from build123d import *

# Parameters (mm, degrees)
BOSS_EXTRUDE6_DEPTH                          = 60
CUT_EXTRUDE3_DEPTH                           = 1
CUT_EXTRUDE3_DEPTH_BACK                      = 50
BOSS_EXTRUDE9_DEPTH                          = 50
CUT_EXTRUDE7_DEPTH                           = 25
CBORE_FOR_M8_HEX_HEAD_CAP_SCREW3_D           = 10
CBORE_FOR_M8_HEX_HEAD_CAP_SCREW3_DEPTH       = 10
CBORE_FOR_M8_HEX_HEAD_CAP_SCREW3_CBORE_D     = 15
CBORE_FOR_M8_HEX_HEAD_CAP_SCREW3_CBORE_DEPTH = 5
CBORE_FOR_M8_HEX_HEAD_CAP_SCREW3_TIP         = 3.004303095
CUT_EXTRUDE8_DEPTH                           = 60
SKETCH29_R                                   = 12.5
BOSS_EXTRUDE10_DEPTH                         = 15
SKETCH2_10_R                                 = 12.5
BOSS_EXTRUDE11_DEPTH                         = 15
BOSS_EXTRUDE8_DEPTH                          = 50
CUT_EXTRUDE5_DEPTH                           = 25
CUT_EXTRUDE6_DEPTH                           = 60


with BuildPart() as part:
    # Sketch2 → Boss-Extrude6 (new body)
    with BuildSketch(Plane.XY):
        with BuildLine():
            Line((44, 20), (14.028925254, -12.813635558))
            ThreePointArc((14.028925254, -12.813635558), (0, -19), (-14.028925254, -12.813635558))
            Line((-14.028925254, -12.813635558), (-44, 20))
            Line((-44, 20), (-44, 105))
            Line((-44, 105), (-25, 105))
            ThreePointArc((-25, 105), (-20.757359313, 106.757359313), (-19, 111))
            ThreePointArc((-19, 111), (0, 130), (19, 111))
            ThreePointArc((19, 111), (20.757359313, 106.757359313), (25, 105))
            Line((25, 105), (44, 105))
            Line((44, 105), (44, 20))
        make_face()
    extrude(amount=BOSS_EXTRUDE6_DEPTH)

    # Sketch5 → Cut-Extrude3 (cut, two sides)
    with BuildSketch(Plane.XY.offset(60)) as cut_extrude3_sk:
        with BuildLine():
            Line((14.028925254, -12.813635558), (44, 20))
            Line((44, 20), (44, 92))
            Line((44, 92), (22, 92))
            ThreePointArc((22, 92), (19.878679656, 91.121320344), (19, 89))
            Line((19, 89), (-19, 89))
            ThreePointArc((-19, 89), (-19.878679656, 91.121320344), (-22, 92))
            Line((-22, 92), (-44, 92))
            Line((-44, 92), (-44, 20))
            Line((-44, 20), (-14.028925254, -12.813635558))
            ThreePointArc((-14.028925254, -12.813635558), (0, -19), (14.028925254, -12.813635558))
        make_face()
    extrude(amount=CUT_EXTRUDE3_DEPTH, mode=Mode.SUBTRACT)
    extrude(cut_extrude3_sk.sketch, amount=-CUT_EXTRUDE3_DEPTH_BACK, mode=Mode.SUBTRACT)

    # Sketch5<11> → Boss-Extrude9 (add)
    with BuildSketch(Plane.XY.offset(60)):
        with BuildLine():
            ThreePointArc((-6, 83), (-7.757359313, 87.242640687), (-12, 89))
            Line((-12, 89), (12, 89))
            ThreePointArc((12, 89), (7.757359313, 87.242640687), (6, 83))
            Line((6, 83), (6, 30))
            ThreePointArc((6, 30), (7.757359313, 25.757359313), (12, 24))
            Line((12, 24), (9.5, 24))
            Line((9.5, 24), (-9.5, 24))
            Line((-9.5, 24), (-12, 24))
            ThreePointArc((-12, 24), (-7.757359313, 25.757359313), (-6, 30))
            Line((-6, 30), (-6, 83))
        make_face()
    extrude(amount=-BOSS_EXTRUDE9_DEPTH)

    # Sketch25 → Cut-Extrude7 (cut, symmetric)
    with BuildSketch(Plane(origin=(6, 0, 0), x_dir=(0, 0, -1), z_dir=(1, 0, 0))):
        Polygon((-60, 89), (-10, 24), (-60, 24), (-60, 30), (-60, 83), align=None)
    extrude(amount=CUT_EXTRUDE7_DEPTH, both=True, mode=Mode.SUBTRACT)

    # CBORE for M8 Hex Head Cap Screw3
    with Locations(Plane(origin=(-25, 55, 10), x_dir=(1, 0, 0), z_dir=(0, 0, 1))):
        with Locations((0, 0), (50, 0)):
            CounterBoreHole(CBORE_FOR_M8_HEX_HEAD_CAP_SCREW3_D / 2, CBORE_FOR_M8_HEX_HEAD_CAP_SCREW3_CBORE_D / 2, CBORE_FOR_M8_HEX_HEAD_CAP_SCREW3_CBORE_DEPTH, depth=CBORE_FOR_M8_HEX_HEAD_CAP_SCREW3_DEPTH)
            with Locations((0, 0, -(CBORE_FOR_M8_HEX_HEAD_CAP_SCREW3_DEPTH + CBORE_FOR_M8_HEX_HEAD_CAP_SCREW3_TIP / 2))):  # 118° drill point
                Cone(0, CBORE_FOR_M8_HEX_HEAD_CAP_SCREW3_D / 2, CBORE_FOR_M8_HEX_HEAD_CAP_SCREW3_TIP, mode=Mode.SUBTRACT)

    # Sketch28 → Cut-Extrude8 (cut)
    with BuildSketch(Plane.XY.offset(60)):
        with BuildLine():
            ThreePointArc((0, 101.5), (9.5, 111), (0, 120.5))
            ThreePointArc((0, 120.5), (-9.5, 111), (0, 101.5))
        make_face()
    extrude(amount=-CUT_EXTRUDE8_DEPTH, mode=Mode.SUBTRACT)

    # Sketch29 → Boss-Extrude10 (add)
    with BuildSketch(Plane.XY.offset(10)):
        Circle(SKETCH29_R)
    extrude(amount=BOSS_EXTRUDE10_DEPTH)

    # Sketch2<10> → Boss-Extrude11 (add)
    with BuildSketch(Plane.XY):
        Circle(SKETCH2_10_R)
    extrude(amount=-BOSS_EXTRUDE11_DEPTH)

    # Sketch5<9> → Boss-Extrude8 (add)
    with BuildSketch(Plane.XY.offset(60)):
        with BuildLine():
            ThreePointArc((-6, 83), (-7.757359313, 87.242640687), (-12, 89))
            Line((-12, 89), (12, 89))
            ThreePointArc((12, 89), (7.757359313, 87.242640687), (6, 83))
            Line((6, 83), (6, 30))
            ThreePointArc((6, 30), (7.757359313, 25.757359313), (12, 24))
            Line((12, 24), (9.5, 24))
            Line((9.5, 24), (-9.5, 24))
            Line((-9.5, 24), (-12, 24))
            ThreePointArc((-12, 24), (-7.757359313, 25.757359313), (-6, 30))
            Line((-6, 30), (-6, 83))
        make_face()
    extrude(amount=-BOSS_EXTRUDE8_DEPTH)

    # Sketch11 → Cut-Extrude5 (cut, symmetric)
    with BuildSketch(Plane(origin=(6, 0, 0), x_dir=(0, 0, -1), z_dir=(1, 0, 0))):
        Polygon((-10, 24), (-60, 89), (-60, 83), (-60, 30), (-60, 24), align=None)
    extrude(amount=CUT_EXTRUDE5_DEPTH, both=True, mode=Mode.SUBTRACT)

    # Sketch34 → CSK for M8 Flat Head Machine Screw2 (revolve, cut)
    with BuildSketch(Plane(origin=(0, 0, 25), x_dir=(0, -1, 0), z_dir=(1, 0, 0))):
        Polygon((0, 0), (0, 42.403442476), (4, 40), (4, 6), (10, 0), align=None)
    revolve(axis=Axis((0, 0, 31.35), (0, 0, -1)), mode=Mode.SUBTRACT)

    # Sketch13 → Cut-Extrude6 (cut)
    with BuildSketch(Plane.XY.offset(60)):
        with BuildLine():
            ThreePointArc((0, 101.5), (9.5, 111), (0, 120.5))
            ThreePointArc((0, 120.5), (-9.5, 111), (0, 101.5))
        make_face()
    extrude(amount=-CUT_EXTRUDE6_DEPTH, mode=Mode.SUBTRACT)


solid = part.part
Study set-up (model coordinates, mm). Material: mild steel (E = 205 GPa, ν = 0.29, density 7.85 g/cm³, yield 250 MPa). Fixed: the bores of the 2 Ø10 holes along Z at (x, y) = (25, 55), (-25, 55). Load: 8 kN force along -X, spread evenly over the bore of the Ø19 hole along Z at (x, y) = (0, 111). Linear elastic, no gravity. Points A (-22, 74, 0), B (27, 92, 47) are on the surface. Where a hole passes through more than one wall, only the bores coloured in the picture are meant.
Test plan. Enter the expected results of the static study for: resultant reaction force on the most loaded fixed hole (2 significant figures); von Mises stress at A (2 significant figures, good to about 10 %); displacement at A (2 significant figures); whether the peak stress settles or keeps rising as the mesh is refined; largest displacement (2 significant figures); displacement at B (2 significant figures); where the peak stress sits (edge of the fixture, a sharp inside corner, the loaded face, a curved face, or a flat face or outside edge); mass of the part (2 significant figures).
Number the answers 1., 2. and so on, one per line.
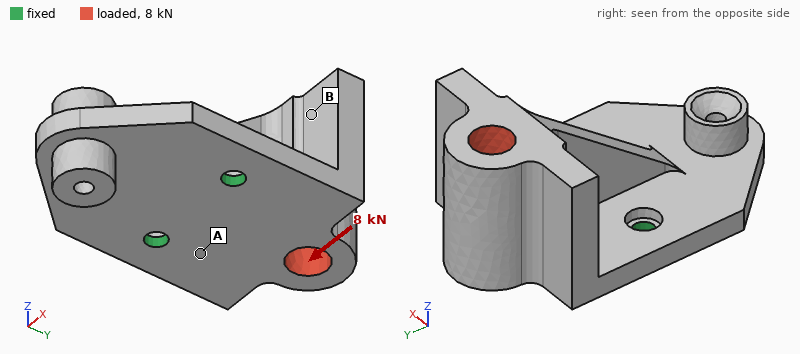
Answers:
1. 10 kN
2. 24 MPa
3. 11 µm
4. keeps rising
5. 72 µm
6. 53 µm
7. edge of the fixture
8. 1.7 kg
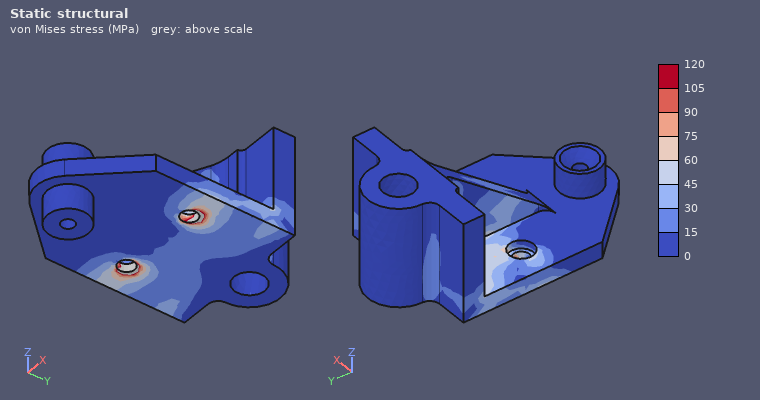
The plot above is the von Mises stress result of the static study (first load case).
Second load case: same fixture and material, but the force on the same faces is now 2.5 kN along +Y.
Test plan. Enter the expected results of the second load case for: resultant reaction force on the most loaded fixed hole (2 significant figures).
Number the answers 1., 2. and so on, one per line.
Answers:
1. 1.3 kN
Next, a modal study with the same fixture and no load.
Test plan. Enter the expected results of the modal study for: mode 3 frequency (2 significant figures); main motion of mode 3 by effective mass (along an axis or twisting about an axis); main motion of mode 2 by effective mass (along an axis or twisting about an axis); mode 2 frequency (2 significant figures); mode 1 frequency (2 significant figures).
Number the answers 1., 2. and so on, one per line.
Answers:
1. 2200 Hz
2. along Z
3. along X
4. 1900 Hz
5. 740 Hz
